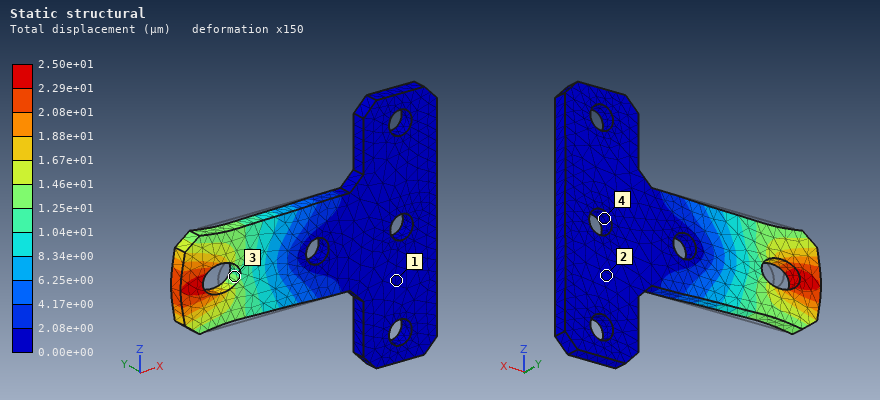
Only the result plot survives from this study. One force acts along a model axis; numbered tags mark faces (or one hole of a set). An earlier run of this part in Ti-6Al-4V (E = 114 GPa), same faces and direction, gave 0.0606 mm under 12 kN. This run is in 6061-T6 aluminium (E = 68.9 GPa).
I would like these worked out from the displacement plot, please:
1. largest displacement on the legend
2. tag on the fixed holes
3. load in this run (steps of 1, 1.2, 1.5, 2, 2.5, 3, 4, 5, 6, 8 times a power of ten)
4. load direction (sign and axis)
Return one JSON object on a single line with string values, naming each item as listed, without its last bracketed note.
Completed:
{"largest displacement on the legend": "2.50e+01 µm", "tag on the fixed holes": "4", "load in this run": "3 kN", "load direction": "-X"}
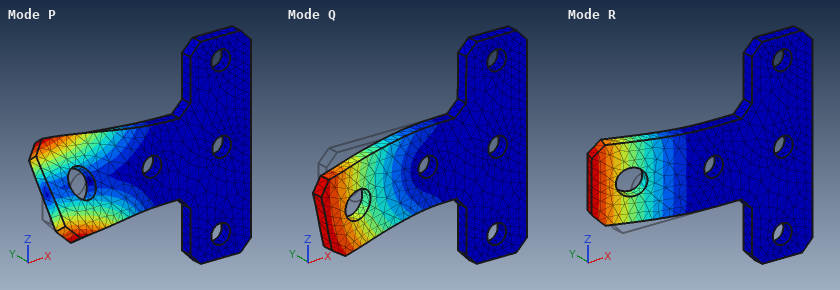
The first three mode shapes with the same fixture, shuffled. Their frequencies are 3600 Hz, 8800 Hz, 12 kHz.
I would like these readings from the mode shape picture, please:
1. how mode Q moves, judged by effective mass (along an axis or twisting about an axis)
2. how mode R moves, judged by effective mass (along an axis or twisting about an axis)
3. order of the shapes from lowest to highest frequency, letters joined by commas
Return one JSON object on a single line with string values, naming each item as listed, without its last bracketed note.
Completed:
{"how mode Q moves, judged by effective mass": "along Z", "how mode R moves, judged by effective mass": "along Y", "order of the shapes from lowest to highest frequency, letters joined by commas": "R, P, Q"}
